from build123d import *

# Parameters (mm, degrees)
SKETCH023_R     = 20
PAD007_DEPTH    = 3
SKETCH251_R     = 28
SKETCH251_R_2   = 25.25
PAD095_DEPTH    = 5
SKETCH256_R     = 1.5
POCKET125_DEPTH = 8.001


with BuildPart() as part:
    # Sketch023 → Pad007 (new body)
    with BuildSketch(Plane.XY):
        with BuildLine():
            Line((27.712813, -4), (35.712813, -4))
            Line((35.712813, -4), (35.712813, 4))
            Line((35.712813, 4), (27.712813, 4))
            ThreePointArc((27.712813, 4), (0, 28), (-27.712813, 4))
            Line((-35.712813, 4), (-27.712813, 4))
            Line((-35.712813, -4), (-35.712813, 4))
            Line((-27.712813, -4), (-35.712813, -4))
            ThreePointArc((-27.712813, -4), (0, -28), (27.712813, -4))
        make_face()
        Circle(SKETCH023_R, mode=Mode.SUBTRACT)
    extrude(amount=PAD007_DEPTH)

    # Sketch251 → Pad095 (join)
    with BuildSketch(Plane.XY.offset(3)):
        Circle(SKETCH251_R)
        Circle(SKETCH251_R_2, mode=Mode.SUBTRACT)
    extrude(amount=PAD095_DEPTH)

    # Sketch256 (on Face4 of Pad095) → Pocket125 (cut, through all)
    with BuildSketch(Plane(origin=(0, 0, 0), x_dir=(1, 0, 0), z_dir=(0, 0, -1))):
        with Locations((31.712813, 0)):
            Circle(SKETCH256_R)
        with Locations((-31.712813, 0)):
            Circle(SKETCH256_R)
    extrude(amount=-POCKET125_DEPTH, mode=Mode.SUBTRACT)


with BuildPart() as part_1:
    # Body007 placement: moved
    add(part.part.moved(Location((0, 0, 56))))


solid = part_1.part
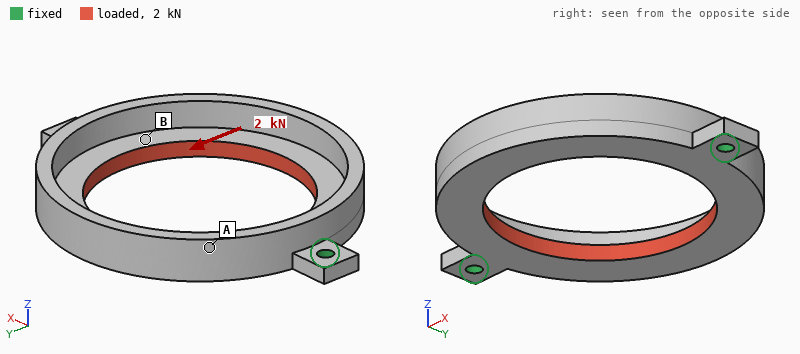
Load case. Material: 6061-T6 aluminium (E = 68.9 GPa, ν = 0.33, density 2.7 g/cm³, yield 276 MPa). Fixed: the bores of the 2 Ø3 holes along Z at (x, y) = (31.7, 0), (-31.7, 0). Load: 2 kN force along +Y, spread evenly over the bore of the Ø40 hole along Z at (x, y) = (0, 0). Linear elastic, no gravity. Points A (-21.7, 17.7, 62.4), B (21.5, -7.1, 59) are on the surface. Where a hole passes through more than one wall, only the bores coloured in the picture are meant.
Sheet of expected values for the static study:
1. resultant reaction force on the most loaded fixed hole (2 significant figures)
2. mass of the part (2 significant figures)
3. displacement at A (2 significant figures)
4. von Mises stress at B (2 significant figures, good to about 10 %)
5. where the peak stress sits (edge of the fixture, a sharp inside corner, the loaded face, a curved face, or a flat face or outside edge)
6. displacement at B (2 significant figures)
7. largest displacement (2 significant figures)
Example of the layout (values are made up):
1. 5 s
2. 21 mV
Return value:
1. 1.0 kN
2. 17 g
3. 15 µm
4. 25 MPa
5. edge of the fixture
6. 16 µm
7. 33 µm
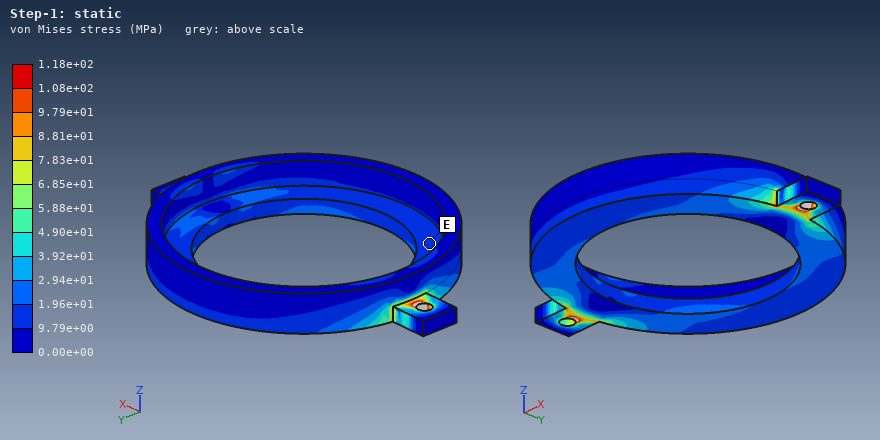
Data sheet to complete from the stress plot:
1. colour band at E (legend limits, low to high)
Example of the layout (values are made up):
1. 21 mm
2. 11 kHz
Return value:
1. 9.79e+00 to 1.96e+01 MPa
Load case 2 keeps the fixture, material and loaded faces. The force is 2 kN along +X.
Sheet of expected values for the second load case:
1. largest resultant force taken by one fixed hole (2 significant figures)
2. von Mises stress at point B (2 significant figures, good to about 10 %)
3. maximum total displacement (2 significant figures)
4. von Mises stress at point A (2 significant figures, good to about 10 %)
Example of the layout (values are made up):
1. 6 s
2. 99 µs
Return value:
1. 1.0 kN
2. 33 MPa
3. 34 µm
4. 9.8 MPa
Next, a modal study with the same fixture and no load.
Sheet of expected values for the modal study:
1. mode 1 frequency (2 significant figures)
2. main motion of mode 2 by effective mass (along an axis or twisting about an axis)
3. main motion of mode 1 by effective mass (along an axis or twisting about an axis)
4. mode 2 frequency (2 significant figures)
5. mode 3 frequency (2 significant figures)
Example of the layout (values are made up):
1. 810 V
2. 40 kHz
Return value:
1. 1800 Hz
2. along Z
3. twisting about X
4. 3100 Hz
5. 6100 Hz
